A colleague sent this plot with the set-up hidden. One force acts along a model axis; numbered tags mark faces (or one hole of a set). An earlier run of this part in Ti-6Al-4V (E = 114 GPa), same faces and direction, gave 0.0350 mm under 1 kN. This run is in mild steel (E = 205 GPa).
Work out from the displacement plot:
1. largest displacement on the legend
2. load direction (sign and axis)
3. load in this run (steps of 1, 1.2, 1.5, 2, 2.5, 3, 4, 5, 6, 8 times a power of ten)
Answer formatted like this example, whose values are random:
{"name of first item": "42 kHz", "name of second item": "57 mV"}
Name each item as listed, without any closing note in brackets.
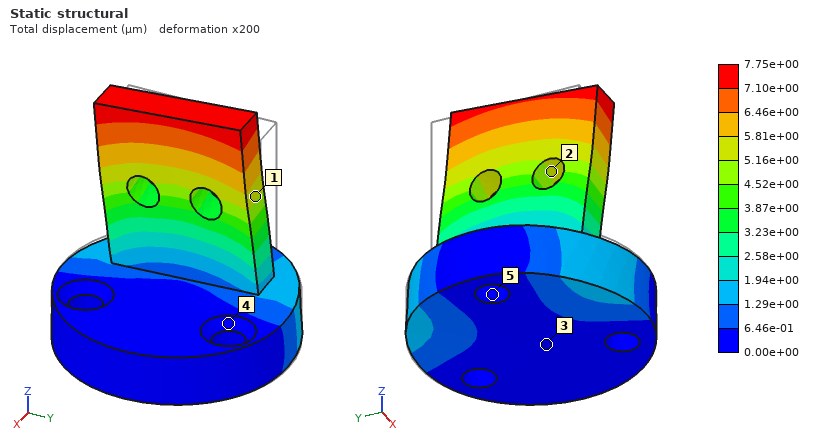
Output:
{"largest displacement on the legend": "7.75e+00 µm", "load direction": "-Y", "load in this run": "400 N"}
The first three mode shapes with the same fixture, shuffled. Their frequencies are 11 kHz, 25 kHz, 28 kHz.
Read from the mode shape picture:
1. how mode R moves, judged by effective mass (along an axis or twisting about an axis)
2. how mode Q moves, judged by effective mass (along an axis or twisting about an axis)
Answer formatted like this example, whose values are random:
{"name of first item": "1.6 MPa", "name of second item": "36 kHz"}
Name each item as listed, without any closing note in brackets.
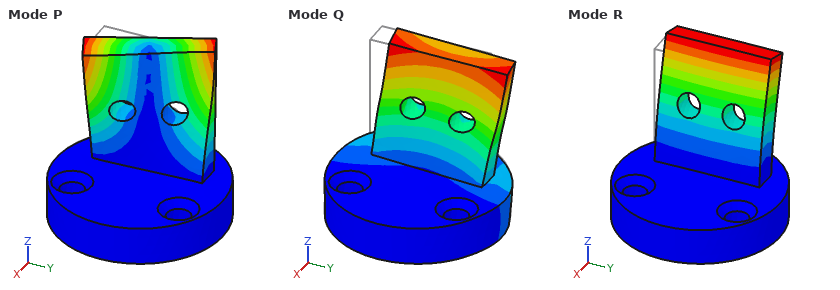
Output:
{"how mode R moves, judged by effective mass": "along X", "how mode Q moves, judged by effective mass": "along Y"}
